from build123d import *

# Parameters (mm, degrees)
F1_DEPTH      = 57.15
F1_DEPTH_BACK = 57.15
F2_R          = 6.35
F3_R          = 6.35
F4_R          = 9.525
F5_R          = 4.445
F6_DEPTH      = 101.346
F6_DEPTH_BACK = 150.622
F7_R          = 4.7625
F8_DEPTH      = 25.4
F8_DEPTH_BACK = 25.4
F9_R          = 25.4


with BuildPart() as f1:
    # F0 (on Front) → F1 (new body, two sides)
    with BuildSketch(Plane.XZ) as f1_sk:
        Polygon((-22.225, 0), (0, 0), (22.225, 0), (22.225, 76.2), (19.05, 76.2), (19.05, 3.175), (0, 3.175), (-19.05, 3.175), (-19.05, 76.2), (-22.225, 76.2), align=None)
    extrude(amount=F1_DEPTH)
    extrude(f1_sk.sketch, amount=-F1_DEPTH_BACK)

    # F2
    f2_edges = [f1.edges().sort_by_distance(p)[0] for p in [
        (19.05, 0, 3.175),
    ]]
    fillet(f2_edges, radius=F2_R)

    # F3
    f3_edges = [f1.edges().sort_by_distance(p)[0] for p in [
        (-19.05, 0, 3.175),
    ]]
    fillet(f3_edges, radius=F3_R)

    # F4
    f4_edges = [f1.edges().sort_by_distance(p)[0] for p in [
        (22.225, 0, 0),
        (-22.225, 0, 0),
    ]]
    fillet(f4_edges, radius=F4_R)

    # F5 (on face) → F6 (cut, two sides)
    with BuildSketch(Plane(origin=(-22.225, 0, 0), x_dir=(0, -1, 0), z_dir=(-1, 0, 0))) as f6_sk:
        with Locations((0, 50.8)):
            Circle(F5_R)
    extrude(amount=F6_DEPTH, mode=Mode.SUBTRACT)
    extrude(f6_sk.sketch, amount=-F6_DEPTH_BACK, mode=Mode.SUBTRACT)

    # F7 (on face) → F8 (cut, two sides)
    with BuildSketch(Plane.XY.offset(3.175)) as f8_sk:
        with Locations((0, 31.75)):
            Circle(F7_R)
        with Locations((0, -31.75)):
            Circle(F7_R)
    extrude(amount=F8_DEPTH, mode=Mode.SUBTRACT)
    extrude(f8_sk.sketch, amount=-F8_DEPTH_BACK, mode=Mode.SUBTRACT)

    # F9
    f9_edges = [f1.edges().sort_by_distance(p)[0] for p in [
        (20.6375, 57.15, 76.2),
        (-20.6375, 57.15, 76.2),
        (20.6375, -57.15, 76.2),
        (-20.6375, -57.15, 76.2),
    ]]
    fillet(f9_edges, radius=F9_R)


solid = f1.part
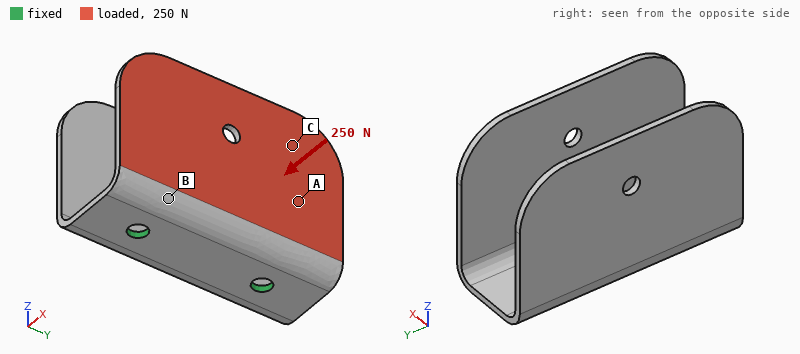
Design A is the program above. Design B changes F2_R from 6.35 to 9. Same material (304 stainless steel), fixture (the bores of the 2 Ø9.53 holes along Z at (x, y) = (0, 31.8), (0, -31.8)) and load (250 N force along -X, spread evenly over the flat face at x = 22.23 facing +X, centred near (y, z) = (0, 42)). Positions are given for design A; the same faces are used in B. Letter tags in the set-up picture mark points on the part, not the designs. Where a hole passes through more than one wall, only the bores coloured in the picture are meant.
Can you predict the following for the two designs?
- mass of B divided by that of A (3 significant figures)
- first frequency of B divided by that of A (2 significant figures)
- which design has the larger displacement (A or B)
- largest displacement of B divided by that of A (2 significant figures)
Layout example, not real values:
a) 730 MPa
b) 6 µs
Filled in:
a) 1.02
b) 1.0
c) A
d) 0.82
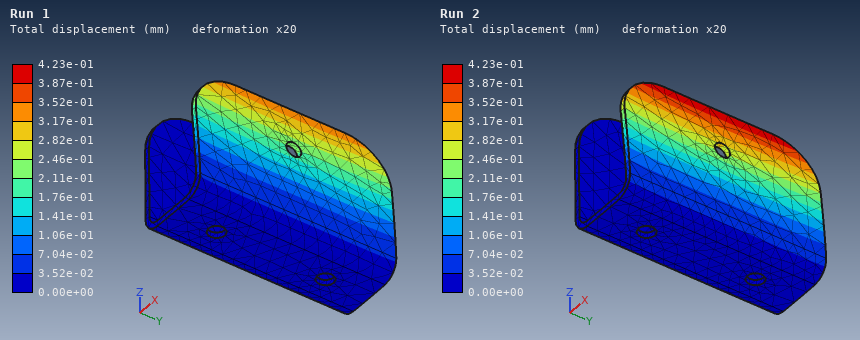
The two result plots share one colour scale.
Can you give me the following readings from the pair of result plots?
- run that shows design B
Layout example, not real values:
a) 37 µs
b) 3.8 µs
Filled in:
a) Run 1
